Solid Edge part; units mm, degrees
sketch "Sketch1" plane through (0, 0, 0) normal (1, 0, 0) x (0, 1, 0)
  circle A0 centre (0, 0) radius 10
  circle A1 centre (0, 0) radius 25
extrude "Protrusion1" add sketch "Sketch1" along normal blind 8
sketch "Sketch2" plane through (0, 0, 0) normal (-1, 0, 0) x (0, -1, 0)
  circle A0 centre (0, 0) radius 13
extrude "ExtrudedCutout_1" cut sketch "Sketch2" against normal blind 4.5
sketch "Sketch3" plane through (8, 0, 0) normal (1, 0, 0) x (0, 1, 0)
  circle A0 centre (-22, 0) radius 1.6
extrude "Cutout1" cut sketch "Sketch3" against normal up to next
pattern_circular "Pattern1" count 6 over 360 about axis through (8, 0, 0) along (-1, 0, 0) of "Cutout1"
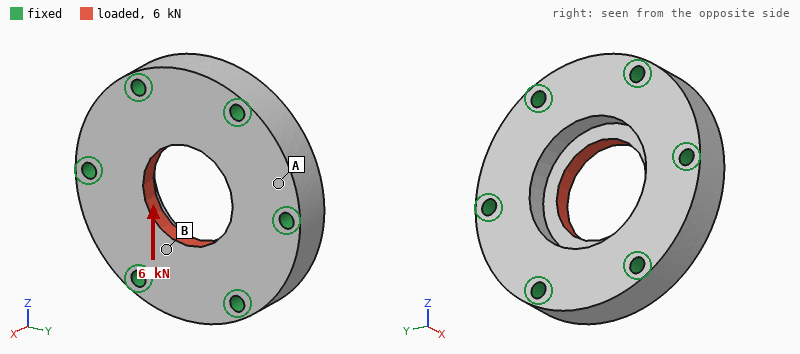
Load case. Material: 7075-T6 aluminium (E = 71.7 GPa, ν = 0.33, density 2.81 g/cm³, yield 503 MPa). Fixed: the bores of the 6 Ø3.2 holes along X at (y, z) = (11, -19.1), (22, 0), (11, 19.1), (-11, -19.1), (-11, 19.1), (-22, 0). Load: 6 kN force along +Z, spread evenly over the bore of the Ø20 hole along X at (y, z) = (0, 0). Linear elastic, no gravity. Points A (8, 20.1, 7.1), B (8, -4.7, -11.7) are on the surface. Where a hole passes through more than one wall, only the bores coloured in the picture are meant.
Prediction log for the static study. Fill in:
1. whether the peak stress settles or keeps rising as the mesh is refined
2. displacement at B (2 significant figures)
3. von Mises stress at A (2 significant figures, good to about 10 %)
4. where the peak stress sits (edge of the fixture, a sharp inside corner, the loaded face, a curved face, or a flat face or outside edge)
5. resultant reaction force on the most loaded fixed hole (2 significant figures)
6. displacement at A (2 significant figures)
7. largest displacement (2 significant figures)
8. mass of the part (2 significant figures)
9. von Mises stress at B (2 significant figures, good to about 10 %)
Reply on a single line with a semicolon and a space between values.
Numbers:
keeps rising; 4.9 µm; 5.3 MPa; edge of the fixture; 1.3 kN; 1.2 µm; 7.0 µm; 33 g; 28 MPa
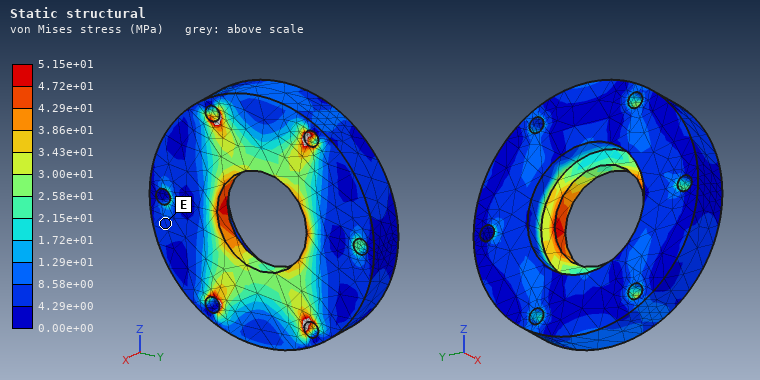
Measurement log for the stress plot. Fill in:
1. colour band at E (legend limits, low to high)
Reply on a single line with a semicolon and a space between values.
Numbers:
4.29e+00 to 8.58e+00 MPa
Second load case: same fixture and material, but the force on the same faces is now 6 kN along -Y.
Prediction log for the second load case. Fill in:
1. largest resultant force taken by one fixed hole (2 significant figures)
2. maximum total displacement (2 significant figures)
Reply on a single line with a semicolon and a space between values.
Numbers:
1.4 kN; 6.6 µm
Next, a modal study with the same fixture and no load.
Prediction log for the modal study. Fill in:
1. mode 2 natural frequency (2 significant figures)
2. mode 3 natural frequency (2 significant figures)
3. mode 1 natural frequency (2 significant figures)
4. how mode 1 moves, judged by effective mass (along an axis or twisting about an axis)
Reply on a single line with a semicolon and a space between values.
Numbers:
44 kHz; 44 kHz; 38 kHz; along X
